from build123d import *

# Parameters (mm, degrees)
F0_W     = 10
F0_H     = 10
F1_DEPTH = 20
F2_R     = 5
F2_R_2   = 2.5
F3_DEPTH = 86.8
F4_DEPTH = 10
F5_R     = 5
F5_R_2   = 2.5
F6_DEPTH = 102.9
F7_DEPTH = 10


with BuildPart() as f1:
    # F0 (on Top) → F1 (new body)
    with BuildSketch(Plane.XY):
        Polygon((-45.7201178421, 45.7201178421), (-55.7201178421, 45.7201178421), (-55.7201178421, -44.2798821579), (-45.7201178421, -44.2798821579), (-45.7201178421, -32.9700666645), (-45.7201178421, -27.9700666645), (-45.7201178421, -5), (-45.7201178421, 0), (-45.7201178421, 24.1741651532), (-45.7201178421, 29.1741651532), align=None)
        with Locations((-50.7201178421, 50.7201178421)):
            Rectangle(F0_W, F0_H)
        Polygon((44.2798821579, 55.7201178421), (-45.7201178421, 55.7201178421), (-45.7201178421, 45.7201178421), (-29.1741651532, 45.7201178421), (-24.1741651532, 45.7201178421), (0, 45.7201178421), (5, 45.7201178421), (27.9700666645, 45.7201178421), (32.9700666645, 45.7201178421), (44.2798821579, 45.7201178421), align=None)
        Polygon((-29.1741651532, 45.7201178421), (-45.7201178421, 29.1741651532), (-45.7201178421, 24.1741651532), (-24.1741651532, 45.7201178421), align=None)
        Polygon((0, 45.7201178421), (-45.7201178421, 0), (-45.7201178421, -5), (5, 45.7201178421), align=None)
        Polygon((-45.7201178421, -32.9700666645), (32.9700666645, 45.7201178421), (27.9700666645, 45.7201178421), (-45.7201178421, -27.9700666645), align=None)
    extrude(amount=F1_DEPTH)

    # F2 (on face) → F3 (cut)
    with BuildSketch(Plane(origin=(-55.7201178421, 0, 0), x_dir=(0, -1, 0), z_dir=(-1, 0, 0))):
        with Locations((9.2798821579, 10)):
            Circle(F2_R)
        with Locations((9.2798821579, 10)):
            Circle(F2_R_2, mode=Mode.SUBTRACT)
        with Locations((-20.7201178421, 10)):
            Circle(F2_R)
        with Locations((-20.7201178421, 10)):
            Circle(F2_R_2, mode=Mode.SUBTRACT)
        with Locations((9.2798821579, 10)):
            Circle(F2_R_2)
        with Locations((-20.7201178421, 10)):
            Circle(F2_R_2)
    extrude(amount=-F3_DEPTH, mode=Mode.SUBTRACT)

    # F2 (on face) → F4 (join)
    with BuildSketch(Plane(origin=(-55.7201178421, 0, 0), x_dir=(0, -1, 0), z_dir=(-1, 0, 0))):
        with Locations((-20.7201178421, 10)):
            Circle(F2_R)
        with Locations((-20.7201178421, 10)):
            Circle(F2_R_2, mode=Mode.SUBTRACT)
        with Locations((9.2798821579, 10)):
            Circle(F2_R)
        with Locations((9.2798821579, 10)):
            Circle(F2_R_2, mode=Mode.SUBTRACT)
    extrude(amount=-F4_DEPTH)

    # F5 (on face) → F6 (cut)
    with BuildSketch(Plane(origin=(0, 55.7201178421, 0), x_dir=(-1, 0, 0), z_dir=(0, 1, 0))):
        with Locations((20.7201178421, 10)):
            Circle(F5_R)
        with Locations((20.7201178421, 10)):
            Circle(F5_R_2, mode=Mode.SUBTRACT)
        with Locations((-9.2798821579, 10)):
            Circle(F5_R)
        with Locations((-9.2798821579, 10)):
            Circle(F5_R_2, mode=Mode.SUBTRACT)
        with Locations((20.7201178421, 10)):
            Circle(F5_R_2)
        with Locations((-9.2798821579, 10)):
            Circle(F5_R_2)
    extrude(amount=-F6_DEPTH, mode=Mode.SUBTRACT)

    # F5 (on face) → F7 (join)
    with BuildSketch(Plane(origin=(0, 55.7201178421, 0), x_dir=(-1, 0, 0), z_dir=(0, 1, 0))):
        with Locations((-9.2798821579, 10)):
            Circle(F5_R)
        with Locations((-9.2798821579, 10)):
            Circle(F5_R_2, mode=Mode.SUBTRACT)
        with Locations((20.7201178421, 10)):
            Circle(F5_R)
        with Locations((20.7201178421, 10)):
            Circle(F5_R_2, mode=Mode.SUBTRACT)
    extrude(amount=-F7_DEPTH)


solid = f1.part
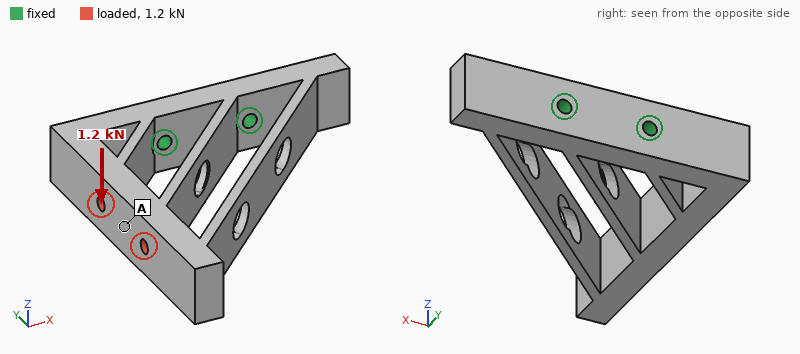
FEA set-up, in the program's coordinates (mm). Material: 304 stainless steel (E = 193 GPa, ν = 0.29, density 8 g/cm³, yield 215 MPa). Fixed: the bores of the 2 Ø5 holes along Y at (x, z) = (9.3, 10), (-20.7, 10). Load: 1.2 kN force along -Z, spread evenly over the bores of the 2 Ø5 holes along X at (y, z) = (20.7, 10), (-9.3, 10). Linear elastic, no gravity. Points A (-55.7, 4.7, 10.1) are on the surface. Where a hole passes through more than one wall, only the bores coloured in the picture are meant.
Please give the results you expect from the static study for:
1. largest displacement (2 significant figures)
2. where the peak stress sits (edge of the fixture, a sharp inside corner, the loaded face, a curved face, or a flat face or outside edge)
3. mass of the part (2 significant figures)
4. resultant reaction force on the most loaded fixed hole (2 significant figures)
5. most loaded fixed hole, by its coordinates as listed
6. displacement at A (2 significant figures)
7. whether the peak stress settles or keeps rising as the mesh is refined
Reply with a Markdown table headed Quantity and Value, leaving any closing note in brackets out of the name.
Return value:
| Quantity | Value |
|---|---|
| largest displacement | 0.16 mm |
| where the peak stress sits | edge of the fixture |
| mass of the part | 400 g |
| resultant reaction force on the most loaded fixed hole | 1.9 kN |
| most loaded fixed hole, by its coordinates as listed | (-20.7, 10) |
| displacement at A | 0.081 mm |
| whether the peak stress settles or keeps rising as the mesh is refined | keeps rising |
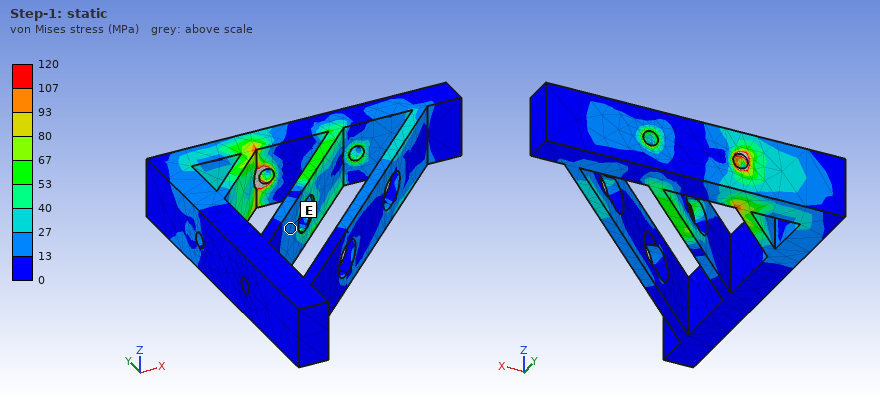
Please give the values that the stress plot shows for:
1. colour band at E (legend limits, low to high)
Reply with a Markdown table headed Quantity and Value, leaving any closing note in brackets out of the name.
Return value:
| Quantity | Value |
|---|---|
| colour band at E | 13 to 27 MPa |
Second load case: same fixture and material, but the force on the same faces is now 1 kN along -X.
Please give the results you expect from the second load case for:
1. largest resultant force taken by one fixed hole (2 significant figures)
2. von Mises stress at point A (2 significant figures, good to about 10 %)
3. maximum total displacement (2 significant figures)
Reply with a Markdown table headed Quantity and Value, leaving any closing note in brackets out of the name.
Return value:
| Quantity | Value |
|---|---|
| largest resultant force taken by one fixed hole | 1.0 kN |
| von Mises stress at point A | 8.3 MPa |
| maximum total displacement | 36 µm |
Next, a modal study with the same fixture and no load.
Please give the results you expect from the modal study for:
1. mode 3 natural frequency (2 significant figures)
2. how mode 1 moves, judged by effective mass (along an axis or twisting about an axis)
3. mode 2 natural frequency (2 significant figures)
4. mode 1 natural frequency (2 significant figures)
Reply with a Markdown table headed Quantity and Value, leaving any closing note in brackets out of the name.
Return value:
| Quantity | Value |
|---|---|
| mode 3 natural frequency | 1900 Hz |
| how mode 1 moves, judged by effective mass | along Z |
| mode 2 natural frequency | 1500 Hz |
| mode 1 natural frequency | 1100 Hz |
